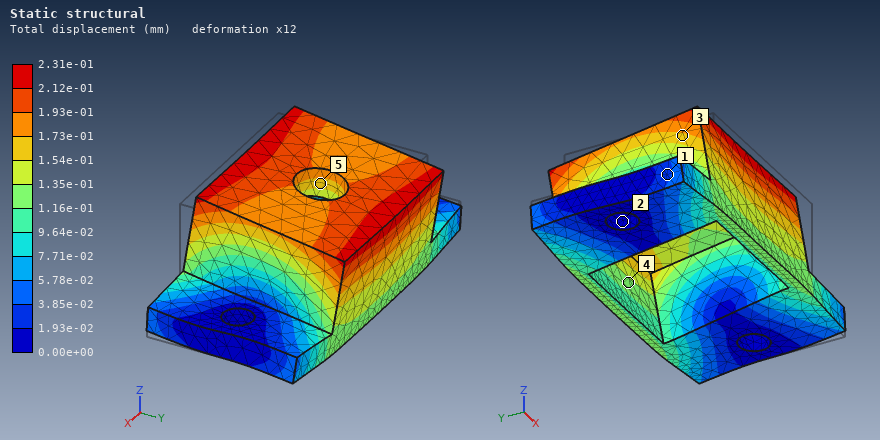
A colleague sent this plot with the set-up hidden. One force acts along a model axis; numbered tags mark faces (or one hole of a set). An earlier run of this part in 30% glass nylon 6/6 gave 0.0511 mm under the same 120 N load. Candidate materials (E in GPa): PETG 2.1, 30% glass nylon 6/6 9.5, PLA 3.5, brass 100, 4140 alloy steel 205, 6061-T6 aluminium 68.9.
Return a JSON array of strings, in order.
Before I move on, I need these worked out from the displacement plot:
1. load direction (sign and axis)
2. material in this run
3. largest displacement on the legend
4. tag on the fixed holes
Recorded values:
["+Y", "PETG", "2.31e-01 mm", "2"]
